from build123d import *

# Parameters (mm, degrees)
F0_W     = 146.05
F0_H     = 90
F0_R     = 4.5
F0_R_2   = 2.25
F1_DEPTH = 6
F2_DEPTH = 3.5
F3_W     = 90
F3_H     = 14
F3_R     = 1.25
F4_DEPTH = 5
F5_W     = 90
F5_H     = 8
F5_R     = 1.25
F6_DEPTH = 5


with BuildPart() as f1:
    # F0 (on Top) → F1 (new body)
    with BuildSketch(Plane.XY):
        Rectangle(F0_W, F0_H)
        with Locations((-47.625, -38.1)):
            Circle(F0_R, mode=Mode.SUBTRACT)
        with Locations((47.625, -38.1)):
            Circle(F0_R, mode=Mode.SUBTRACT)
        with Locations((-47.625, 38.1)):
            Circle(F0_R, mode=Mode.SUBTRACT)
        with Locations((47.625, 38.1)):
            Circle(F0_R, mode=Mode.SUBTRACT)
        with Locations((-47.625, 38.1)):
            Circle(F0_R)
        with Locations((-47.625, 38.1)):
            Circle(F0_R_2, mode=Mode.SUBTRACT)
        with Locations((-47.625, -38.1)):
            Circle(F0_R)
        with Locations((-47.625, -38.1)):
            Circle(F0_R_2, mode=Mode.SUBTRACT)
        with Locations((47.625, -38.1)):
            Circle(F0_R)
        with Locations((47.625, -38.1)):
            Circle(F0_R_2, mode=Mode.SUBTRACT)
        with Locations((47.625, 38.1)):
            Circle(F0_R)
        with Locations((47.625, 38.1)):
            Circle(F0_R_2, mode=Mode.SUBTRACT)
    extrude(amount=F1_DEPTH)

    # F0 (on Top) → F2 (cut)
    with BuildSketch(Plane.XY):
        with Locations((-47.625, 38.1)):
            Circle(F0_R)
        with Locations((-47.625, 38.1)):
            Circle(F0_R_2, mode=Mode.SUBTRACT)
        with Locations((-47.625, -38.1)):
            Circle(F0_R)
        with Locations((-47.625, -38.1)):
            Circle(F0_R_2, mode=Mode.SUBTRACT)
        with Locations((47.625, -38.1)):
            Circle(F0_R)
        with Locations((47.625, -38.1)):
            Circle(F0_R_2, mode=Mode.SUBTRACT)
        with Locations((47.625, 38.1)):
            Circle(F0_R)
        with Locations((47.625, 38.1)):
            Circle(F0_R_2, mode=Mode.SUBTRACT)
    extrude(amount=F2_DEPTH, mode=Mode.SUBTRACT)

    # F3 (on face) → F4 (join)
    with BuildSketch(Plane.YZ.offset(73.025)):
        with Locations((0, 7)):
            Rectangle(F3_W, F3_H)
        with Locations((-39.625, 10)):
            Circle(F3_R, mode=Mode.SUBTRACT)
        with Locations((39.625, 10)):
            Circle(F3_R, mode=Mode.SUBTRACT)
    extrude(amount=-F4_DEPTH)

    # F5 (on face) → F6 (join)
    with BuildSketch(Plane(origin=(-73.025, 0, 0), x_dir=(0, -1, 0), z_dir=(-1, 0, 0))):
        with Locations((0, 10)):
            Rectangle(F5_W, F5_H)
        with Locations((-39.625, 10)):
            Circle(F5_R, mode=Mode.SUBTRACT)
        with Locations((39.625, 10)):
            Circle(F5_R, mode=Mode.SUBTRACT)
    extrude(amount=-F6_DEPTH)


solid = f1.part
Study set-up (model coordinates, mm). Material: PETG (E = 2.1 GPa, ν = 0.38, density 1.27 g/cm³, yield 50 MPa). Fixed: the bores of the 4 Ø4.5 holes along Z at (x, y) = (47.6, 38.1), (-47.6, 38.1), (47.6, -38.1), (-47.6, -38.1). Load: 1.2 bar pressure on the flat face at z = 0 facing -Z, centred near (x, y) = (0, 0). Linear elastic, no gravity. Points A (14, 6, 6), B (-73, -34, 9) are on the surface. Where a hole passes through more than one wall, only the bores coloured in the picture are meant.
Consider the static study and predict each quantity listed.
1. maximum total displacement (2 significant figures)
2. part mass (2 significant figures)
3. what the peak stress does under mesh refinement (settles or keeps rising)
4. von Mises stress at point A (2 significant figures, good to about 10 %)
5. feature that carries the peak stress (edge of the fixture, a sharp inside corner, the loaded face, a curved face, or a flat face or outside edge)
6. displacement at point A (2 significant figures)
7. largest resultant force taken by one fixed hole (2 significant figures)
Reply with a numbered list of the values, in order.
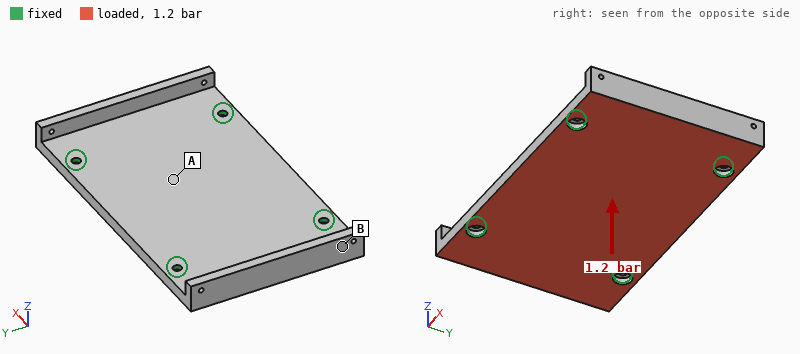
1. 1.6 mm
2. 110 g
3. keeps rising
4. 8.0 MPa
5. edge of the fixture
6. 1.5 mm
7. 560 N
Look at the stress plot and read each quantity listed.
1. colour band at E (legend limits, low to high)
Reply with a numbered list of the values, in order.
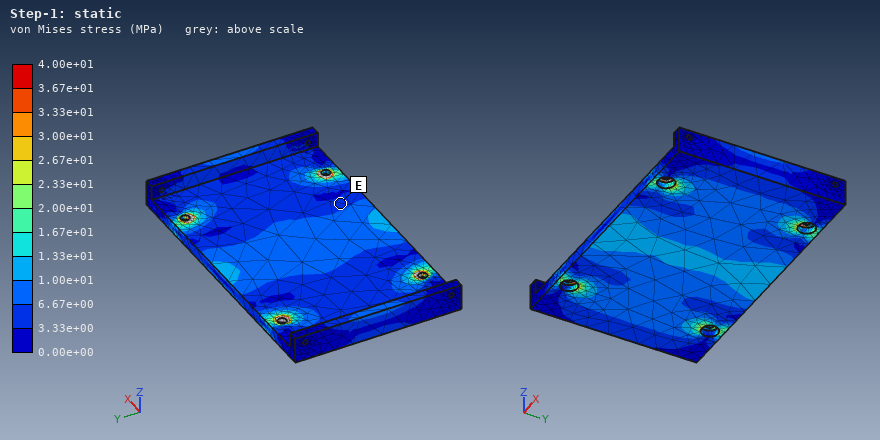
1. 3.33e+00 to 6.67e+00 MPa
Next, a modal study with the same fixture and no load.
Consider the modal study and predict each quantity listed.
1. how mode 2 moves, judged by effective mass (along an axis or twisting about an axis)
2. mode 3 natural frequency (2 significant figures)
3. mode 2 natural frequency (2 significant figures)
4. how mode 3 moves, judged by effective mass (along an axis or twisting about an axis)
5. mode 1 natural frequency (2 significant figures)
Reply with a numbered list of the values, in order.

1. twisting about Y
2. 730 Hz
3. 700 Hz
4. along Z
5. 510 Hz
